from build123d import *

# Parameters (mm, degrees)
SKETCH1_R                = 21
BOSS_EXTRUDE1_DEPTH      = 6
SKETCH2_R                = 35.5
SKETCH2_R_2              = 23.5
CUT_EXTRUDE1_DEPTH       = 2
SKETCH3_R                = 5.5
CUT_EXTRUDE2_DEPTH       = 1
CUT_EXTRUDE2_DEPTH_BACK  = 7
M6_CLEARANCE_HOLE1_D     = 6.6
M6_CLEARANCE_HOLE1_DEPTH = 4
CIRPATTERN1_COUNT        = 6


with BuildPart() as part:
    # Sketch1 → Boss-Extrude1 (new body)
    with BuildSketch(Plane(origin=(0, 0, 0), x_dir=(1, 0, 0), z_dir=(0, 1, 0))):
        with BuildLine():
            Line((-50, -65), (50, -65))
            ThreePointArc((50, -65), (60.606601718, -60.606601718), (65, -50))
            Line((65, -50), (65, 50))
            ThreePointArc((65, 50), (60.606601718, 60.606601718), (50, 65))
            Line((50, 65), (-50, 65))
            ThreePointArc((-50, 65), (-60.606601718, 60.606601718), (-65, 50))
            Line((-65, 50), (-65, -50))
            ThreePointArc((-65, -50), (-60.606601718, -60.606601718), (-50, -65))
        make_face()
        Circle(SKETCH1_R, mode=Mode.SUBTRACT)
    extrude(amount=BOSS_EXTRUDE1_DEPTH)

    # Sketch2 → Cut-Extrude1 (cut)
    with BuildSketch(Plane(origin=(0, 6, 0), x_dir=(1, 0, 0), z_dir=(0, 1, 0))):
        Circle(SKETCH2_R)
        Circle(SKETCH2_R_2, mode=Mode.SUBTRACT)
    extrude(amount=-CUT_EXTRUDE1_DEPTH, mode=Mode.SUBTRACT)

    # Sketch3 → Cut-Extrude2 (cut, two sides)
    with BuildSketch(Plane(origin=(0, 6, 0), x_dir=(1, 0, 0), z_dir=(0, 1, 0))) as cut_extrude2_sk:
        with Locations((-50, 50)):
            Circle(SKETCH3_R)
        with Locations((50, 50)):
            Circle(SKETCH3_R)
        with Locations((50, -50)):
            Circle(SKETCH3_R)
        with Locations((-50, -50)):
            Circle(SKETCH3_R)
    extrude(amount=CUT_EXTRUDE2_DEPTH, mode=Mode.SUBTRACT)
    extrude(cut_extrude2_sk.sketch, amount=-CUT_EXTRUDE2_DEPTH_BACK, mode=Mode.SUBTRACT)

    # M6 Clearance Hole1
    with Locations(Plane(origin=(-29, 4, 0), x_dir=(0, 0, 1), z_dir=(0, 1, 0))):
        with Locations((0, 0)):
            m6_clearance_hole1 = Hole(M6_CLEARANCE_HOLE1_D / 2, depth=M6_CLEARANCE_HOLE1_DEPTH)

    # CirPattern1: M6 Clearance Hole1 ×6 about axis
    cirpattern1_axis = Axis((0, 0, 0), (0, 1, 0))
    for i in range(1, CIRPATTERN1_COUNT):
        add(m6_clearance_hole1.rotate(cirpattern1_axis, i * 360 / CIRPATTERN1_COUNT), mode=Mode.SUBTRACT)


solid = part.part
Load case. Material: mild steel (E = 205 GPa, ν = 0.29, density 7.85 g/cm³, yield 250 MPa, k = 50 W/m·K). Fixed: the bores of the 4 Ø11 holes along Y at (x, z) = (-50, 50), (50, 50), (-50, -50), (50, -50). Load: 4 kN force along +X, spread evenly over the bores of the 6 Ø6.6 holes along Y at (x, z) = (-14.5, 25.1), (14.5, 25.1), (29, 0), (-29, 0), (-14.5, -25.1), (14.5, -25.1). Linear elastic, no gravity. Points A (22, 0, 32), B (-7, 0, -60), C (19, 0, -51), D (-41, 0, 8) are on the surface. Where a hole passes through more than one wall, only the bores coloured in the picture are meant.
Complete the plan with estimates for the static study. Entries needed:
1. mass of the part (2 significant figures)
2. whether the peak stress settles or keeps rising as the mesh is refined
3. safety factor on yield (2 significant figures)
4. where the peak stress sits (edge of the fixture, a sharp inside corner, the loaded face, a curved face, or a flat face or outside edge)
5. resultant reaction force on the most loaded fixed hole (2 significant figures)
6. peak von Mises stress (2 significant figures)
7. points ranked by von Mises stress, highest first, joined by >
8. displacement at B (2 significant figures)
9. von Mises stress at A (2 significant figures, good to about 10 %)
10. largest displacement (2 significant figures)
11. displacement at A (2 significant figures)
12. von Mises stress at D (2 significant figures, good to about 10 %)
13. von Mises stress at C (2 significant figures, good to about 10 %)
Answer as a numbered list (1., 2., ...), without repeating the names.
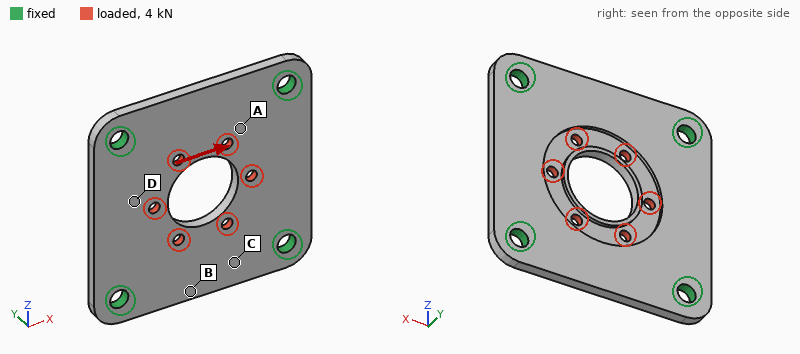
1. 660 g
2. settles
3. 12
4. the loaded face
5. 1.1 kN
6. 20 MPa
7. A > D > C > B
8. 0.48 µm
9. 6.7 MPa
10. 2.5 µm
11. 1.0 µm
12. 4.7 MPa
13. 3.1 MPa
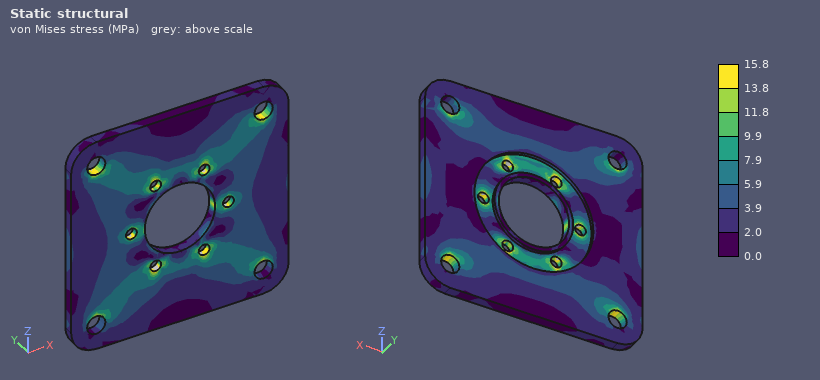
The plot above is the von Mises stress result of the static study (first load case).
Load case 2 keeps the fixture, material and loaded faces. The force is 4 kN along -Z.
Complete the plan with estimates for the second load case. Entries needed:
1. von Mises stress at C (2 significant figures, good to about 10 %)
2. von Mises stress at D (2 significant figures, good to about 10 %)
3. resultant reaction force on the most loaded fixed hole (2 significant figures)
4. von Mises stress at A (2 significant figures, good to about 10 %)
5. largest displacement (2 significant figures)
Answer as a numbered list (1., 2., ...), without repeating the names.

1. 3.6 MPa
2. 4.0 MPa
3. 1.1 kN
4. 7.5 MPa
5. 2.3 µm
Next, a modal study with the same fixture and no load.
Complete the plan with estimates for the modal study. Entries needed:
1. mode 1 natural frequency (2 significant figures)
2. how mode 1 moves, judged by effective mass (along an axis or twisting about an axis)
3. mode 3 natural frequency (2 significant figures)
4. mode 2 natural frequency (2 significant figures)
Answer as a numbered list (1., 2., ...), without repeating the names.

1. 2700 Hz
2. along Y
3. 3600 Hz
4. 3600 Hz
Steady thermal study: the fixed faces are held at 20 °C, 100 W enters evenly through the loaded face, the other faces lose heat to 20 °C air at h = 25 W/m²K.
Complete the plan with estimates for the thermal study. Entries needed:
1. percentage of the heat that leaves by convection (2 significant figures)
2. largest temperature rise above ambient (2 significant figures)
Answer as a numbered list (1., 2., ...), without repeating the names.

1. 26 %
2. 77 K
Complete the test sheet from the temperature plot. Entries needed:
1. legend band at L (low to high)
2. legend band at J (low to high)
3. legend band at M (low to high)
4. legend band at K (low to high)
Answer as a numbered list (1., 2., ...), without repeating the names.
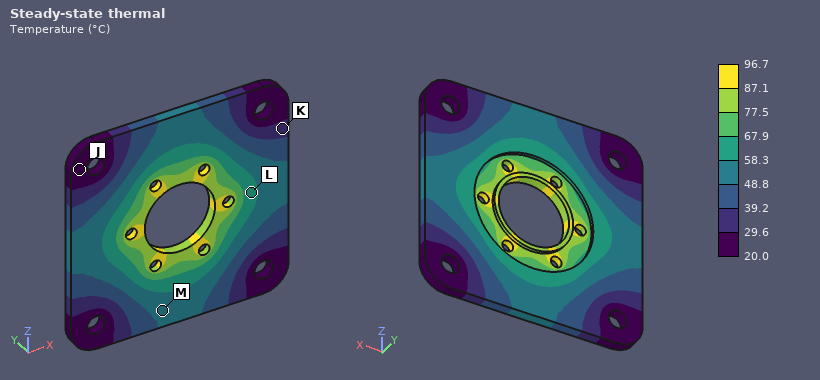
1. 58.3 to 67.9 °C
2. 20.0 to 29.6 °C
3. 48.8 to 58.3 °C
4. 29.6 to 39.2 °C
